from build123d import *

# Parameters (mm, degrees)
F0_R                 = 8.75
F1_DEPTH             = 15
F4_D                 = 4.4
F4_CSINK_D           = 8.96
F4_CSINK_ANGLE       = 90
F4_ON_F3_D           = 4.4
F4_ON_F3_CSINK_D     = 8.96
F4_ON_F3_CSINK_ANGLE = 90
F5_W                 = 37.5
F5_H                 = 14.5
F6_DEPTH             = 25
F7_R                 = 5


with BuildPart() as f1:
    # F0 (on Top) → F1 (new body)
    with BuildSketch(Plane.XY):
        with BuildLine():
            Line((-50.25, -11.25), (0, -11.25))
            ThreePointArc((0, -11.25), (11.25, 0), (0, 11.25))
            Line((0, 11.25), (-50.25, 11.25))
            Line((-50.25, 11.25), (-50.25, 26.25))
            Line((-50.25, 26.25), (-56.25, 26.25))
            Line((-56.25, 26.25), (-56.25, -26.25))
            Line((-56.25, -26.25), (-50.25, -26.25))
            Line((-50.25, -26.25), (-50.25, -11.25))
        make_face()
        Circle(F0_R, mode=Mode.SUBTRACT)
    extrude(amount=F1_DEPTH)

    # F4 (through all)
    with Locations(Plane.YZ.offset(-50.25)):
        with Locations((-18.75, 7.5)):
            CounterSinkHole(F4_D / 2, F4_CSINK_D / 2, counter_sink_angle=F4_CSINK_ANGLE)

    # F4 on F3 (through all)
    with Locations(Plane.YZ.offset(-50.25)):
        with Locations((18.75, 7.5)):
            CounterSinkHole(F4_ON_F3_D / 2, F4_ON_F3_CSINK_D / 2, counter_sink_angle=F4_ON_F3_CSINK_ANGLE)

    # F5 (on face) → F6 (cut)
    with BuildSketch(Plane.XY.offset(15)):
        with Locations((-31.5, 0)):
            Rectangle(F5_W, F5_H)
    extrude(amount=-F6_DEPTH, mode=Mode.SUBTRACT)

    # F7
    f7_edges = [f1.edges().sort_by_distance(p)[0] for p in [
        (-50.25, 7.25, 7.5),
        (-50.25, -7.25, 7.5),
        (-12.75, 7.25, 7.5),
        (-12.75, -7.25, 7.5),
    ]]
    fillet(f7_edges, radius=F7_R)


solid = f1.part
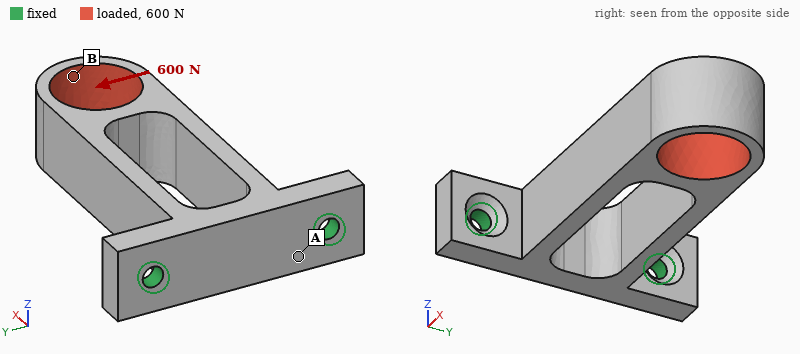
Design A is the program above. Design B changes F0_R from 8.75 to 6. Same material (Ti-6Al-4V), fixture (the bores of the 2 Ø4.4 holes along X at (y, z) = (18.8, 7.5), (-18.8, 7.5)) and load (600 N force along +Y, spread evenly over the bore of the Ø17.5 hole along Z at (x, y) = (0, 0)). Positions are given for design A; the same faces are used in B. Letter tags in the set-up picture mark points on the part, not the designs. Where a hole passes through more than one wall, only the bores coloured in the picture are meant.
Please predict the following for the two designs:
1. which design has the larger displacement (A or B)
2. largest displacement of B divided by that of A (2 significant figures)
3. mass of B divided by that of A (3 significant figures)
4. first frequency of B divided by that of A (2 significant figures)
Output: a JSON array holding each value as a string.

["A", "0.90", "1.15", "0.83"]
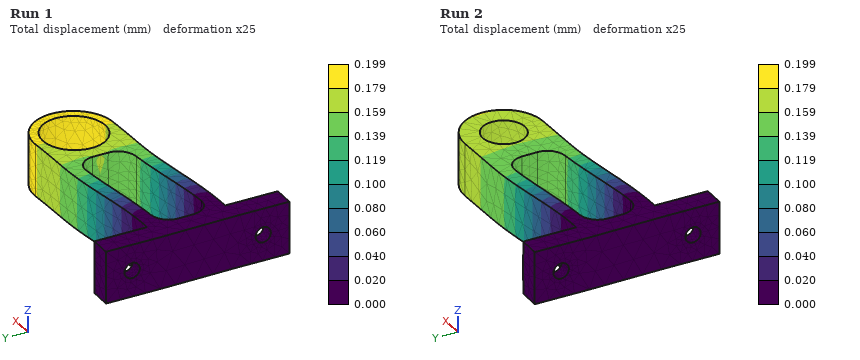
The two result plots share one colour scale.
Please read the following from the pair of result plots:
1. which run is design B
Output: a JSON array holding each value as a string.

["Run 2"]
